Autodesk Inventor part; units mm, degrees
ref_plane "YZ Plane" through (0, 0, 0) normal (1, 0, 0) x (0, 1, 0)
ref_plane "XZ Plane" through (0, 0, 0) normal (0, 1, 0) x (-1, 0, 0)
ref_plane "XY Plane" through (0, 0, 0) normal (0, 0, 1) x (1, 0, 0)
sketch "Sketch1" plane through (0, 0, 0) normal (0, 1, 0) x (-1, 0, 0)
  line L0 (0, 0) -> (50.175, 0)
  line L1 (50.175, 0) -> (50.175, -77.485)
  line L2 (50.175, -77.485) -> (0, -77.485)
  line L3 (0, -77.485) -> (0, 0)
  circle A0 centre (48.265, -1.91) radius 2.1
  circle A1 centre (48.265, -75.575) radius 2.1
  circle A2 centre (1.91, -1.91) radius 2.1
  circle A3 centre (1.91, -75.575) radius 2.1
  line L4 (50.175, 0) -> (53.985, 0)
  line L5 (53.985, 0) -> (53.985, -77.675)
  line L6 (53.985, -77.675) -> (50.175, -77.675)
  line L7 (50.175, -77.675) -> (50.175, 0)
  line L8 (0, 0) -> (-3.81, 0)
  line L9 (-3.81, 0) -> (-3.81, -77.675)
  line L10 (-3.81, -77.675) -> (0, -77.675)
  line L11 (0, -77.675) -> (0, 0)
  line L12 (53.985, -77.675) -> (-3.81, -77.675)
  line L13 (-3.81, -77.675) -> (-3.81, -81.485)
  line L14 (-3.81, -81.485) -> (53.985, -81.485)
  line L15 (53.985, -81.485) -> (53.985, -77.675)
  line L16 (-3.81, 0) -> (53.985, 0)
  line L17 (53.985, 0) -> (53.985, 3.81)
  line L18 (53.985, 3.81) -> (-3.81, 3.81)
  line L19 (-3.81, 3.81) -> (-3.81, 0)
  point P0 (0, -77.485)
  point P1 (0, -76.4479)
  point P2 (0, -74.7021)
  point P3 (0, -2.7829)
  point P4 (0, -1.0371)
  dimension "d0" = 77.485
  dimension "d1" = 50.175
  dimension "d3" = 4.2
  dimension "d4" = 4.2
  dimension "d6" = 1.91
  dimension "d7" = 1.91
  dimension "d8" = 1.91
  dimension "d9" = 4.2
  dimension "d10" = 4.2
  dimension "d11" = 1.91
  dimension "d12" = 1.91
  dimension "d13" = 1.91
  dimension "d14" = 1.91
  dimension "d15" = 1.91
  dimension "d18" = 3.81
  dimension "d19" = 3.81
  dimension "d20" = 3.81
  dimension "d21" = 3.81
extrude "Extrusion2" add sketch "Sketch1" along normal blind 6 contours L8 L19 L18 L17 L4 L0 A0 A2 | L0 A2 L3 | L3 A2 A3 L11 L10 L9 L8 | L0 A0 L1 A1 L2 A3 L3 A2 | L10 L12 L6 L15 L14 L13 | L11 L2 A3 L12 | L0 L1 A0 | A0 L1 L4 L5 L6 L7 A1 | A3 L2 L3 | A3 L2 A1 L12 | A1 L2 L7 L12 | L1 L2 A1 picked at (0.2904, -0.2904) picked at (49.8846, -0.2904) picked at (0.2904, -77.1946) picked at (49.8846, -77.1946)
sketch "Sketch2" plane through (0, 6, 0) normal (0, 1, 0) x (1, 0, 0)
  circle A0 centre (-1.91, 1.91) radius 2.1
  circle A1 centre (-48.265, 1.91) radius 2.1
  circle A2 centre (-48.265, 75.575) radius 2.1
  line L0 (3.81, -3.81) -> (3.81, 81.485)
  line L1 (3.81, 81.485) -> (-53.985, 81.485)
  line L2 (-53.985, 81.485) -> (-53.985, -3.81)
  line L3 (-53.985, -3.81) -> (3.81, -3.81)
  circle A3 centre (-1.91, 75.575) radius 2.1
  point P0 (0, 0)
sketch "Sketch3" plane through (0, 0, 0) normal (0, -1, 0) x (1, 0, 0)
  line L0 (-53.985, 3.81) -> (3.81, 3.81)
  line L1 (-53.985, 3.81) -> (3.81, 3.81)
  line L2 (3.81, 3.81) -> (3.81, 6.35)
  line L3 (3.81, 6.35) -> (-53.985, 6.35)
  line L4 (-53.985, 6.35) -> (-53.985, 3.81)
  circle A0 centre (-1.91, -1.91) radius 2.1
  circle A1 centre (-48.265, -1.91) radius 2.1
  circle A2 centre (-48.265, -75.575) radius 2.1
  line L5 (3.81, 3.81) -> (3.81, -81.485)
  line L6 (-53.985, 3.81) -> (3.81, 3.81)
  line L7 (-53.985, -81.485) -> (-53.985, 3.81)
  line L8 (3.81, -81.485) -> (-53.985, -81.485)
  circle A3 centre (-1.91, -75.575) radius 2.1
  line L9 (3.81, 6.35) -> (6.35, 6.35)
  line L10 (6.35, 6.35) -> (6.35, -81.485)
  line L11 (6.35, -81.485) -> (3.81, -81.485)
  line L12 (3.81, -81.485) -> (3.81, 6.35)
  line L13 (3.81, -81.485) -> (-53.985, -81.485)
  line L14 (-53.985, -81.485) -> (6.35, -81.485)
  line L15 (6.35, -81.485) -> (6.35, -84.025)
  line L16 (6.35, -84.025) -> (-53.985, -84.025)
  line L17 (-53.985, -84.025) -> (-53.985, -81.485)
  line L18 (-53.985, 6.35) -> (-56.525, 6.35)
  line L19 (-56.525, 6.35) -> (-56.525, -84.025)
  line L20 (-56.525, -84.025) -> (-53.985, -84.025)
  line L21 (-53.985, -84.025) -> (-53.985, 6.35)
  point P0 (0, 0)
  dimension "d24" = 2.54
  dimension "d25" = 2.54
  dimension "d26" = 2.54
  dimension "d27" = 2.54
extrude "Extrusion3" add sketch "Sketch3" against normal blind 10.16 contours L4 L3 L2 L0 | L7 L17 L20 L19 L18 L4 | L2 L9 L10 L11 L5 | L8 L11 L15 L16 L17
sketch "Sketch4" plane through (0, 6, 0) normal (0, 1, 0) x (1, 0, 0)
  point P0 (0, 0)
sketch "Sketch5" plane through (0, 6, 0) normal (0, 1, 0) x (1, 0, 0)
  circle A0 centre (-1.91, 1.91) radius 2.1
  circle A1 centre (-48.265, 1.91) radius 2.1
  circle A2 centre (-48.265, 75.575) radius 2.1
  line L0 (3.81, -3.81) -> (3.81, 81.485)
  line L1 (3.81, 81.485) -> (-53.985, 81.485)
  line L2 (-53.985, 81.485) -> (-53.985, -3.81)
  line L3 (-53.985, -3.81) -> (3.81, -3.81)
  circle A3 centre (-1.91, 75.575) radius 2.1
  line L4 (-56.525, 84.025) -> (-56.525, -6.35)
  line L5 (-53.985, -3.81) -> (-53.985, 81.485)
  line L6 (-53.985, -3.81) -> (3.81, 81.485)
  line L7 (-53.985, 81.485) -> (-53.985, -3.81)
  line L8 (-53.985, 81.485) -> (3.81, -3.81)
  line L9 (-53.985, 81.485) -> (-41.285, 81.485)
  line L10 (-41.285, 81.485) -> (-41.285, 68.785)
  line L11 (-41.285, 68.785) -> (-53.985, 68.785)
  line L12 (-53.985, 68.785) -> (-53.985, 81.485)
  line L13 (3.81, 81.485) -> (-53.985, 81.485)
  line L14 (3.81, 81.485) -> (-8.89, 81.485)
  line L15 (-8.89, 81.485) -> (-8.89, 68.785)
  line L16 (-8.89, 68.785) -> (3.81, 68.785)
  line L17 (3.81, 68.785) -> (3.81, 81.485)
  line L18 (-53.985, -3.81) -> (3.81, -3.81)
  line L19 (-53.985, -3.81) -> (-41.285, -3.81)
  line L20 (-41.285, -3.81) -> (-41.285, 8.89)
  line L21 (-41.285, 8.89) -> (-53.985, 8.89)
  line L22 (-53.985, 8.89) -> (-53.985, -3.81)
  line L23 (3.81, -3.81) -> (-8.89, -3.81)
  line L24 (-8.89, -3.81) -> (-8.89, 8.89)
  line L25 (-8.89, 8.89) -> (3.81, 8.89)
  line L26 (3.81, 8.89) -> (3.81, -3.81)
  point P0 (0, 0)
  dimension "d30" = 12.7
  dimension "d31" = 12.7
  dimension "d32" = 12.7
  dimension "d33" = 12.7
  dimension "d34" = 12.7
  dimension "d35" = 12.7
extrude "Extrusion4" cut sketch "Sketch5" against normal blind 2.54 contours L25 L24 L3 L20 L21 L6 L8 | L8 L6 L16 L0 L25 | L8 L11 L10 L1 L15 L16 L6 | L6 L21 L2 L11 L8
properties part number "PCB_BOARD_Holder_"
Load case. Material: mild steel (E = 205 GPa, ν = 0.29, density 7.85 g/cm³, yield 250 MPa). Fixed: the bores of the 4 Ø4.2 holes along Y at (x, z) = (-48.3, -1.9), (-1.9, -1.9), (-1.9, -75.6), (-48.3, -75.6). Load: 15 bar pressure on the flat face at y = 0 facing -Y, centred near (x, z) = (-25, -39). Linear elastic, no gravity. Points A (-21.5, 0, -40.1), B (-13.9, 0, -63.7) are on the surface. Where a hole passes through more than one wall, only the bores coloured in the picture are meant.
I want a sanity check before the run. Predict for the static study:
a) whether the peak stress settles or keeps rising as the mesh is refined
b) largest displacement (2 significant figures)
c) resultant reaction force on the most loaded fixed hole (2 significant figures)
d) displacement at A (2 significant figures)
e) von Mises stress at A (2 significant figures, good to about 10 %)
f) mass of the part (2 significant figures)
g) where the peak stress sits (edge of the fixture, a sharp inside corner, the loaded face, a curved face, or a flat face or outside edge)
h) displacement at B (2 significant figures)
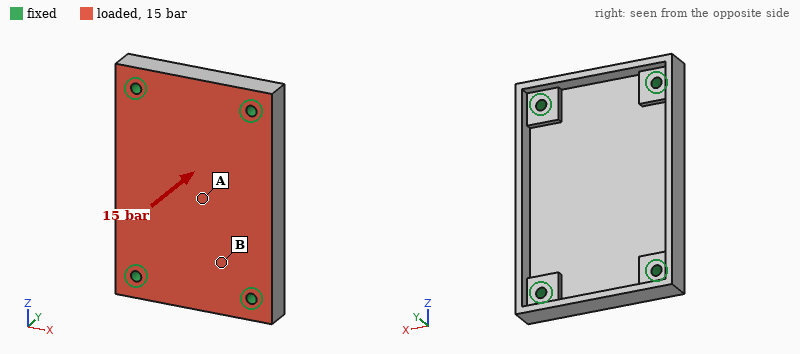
keeps rising
0.11 mm
2.3 kN
0.11 mm
110 MPa
200 g
edge of the fixture
0.038 mm
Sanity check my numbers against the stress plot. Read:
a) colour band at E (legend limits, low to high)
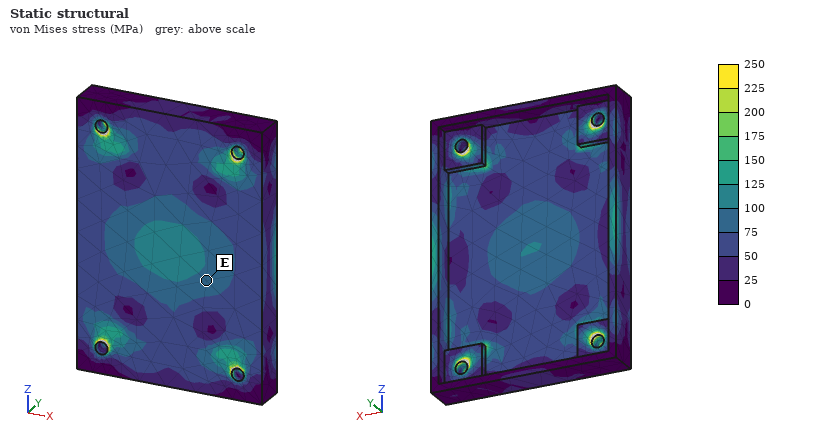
75 to 100 MPa
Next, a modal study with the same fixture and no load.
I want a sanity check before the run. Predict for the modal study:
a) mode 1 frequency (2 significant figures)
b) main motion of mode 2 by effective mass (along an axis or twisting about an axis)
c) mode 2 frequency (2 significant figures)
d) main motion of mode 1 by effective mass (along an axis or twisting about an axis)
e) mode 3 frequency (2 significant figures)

4500 Hz
twisting about Z
6800 Hz
along Y
8400 Hz
